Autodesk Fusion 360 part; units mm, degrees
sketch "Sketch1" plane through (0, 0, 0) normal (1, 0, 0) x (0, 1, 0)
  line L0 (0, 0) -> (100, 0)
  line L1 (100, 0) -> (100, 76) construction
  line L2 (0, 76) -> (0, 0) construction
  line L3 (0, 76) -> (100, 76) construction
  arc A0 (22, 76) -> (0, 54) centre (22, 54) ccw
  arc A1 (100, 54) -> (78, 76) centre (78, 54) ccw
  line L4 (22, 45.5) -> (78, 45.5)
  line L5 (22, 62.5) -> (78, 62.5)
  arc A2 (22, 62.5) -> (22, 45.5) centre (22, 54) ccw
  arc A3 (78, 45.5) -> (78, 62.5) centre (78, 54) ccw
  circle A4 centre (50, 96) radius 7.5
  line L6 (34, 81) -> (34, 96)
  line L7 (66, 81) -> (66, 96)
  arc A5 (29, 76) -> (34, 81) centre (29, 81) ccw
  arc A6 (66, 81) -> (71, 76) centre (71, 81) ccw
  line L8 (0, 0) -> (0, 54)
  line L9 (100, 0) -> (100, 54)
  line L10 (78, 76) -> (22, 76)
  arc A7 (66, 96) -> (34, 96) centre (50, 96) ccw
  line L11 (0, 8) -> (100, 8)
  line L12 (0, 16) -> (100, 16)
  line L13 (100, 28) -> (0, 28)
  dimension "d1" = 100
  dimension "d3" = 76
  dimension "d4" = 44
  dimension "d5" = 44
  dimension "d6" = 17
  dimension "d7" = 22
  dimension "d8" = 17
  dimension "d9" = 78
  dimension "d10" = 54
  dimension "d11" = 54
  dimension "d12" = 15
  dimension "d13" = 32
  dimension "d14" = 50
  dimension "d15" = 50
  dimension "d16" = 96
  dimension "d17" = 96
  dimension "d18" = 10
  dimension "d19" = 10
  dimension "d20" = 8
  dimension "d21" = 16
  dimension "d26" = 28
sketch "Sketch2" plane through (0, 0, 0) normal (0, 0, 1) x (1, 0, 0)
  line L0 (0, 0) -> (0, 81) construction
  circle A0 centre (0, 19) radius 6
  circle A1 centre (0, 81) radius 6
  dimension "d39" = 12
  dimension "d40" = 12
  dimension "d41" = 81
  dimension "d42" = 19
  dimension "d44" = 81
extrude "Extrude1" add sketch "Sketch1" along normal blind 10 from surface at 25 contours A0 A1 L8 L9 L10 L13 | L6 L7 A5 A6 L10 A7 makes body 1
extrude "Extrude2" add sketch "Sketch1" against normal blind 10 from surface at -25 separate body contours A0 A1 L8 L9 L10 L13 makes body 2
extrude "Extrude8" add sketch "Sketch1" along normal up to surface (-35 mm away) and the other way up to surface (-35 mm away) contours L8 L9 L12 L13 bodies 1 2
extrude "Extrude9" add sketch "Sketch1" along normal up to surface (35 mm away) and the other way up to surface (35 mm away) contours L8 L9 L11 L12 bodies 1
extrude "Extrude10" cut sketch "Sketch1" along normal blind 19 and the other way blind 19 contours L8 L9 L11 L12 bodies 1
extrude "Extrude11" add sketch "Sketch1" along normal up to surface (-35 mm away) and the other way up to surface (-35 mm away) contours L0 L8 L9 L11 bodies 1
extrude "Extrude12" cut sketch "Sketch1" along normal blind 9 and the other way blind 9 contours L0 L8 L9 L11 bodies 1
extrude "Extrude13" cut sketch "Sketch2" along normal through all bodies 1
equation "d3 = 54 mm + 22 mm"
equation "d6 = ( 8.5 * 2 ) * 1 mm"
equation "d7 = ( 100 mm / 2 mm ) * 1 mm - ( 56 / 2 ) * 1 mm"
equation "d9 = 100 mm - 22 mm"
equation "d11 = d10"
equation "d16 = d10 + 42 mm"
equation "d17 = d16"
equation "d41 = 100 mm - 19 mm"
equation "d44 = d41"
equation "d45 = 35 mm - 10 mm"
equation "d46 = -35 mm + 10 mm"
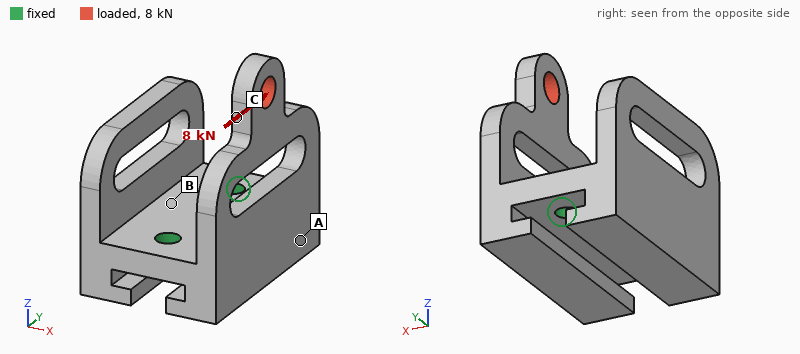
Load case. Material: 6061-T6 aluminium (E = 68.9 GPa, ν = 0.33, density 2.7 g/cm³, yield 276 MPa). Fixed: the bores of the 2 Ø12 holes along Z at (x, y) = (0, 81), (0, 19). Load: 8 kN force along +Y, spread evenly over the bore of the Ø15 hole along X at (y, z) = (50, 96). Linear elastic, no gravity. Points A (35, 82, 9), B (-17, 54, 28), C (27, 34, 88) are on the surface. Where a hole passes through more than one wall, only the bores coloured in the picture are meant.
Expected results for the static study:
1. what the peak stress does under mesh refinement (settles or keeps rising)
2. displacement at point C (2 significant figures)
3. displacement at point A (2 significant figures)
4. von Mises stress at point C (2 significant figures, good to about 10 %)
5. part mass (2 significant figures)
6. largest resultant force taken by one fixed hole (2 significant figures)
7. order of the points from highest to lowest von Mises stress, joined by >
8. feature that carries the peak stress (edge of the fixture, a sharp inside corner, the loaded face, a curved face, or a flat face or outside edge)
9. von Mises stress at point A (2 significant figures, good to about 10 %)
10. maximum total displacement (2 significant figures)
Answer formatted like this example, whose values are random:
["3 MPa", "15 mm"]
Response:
["keeps rising", "0.33 mm", "0.087 mm", "83 MPa", "610 g", "9.7 kN", "C > A > B", "edge of the fixture", "42 MPa", "0.49 mm"]
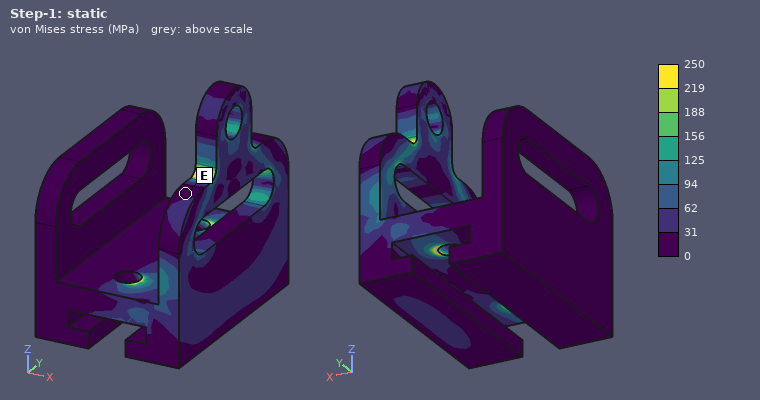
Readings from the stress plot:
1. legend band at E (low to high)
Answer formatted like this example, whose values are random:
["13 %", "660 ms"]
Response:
["0 to 31 MPa"]
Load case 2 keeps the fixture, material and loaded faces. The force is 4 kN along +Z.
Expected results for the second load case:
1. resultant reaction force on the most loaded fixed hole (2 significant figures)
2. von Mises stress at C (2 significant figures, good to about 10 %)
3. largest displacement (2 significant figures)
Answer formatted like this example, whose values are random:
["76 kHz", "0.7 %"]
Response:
["2.0 kN", "14 MPa", "0.19 mm"]
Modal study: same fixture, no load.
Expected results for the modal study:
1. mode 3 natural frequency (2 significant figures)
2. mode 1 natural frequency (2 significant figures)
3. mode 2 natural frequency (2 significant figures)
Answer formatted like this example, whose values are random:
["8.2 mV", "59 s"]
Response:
["3000 Hz", "1000 Hz", "1800 Hz"]
